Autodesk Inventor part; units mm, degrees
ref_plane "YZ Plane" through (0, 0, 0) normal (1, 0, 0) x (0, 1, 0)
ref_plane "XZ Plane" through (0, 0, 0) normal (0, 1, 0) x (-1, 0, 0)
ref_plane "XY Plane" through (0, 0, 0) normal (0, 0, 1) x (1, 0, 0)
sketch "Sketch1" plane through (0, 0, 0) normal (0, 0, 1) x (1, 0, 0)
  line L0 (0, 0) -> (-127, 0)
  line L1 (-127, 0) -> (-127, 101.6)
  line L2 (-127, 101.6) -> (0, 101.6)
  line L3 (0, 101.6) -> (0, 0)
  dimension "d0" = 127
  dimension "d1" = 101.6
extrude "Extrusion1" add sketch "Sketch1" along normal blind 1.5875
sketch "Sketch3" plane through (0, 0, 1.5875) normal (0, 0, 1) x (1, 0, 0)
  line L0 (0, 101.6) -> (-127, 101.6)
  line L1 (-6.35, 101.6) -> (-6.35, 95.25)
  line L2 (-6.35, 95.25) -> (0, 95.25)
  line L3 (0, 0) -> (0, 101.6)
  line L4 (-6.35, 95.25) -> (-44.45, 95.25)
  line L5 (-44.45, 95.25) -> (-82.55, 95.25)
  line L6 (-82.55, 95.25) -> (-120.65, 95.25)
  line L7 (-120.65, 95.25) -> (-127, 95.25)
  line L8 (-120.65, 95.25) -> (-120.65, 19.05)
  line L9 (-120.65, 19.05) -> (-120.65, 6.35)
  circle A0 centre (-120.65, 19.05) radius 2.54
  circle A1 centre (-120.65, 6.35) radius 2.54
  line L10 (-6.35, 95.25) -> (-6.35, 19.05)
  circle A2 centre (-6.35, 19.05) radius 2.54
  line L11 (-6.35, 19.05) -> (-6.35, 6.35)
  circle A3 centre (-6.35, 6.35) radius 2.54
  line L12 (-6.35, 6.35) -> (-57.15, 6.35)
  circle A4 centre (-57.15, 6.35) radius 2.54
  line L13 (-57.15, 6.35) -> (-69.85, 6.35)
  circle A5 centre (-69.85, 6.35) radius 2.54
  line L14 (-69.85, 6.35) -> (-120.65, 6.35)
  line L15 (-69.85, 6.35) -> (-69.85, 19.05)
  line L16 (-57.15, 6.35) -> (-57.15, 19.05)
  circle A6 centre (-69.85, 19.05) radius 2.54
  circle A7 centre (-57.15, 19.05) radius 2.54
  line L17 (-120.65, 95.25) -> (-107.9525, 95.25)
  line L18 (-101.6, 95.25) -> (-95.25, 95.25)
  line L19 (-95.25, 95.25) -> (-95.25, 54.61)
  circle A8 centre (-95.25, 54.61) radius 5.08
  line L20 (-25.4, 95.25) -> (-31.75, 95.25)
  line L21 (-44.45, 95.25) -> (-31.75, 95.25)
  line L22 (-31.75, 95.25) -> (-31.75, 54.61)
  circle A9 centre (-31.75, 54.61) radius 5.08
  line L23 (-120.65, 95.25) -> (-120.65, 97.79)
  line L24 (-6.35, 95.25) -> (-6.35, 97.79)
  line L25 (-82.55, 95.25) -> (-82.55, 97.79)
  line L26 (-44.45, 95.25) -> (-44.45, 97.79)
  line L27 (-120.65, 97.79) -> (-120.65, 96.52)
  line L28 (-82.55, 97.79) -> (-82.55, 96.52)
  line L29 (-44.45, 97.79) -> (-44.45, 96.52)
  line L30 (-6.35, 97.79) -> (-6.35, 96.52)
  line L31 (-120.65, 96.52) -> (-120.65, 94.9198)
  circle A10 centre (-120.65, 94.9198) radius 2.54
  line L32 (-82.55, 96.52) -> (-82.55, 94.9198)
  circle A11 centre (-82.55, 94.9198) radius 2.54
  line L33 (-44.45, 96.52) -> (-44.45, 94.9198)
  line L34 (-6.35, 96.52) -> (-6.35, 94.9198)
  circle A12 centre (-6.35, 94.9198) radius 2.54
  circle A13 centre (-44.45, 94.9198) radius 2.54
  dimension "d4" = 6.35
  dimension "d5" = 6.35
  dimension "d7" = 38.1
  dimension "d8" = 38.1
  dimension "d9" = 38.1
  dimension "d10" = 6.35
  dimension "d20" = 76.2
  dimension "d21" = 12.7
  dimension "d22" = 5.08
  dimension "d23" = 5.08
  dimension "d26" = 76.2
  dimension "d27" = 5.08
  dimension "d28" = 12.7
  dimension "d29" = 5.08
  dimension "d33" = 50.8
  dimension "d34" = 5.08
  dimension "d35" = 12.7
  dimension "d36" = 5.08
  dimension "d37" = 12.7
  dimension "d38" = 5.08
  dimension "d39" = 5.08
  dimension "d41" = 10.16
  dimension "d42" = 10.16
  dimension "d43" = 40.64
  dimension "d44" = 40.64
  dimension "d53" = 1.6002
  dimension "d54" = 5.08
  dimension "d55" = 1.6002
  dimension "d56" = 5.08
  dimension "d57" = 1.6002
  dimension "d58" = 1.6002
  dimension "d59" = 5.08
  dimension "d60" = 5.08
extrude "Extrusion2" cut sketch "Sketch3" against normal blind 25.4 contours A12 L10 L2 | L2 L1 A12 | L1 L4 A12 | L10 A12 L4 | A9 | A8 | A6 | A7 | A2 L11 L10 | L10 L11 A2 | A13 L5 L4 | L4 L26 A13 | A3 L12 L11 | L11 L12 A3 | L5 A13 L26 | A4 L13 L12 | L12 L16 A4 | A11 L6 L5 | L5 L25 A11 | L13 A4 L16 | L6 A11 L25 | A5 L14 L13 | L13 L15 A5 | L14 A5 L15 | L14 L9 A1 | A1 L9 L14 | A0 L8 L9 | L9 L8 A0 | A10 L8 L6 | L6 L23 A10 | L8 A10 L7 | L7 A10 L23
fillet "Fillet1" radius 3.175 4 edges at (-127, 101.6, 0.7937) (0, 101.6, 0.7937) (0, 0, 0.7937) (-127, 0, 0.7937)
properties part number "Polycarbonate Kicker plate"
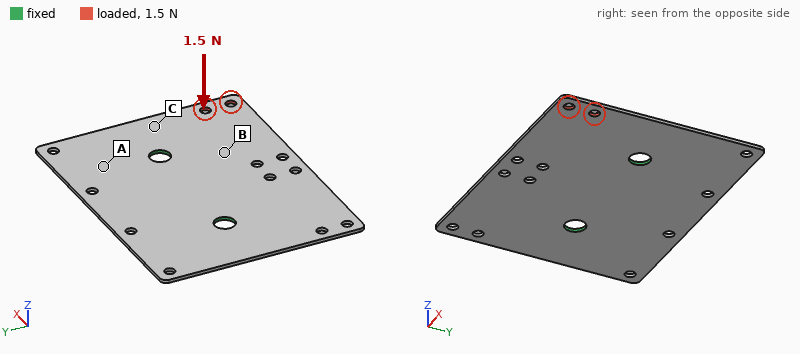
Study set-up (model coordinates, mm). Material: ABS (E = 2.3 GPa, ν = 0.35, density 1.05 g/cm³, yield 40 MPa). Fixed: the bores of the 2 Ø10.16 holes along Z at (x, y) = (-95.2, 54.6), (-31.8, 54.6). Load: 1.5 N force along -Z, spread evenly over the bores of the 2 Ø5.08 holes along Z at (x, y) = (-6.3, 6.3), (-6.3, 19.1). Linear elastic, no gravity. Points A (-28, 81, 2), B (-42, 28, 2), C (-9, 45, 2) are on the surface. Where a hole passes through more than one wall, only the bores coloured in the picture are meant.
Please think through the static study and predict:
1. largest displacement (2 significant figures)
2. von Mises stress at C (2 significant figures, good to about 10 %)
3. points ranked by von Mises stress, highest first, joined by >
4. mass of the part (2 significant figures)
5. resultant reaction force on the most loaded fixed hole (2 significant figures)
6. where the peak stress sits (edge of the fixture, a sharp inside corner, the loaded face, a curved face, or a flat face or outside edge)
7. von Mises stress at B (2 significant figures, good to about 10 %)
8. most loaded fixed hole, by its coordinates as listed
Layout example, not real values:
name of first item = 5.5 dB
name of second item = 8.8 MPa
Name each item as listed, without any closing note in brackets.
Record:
largest displacement = 1.5 mm
von Mises stress at C = 1.7 MPa
points ranked by von Mises stress, highest first, joined by > = C > B > A
mass of the part = 21 g
resultant reaction force on the most loaded fixed hole = 1.7 N
where the peak stress sits = a flat face or outside edge
von Mises stress at B = 1.2 MPa
most loaded fixed hole, by its coordinates as listed = (-31.8, 54.6)
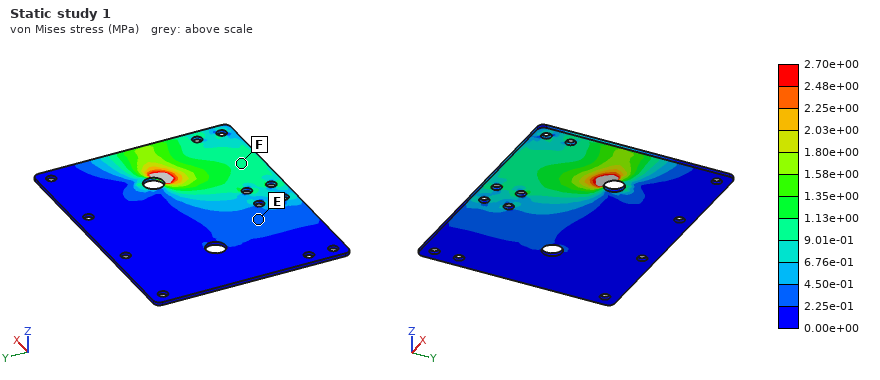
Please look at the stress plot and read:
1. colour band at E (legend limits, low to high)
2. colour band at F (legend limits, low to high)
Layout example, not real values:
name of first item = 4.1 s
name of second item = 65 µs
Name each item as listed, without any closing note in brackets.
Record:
colour band at E = 2.25e-01 to 4.50e-01 MPa
colour band at F = 9.01e-01 to 1.13e+00 MPa
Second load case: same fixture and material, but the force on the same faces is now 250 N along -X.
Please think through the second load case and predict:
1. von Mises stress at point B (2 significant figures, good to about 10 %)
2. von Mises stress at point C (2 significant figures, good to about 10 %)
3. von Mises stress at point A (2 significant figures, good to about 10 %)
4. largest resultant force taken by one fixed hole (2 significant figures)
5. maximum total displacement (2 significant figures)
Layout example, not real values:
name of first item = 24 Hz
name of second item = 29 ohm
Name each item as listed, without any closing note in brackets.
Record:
von Mises stress at point B = 4.0 MPa
von Mises stress at point C = 2.0 MPa
von Mises stress at point A = 1.1 MPa
largest resultant force taken by one fixed hole = 200 N
maximum total displacement = 0.28 mm
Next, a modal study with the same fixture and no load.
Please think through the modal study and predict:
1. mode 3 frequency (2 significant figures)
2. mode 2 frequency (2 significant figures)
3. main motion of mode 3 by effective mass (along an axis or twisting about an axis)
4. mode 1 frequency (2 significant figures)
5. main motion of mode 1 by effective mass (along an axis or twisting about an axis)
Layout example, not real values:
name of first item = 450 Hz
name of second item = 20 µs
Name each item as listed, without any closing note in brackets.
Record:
mode 3 frequency = 190 Hz
mode 2 frequency = 180 Hz
main motion of mode 3 by effective mass = along Z
mode 1 frequency = 140 Hz
main motion of mode 1 by effective mass = along Z
